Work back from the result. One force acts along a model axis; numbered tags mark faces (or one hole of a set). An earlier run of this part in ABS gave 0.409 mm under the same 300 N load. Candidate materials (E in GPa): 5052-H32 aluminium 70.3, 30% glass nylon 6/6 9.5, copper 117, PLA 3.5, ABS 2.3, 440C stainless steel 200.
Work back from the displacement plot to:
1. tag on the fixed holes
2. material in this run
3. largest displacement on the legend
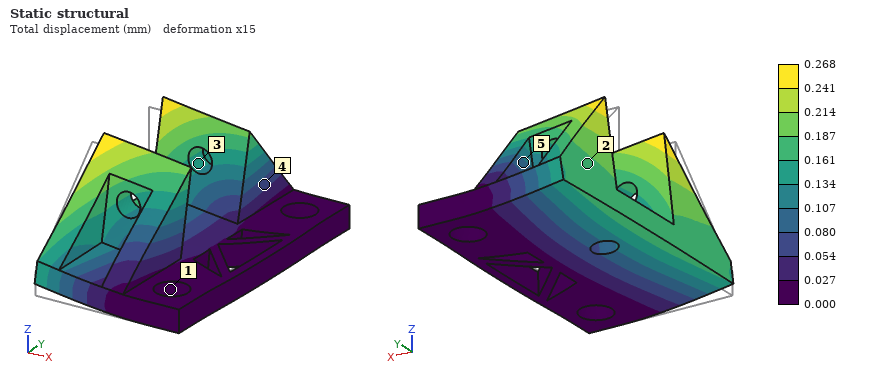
1
PLA
0.268 mm
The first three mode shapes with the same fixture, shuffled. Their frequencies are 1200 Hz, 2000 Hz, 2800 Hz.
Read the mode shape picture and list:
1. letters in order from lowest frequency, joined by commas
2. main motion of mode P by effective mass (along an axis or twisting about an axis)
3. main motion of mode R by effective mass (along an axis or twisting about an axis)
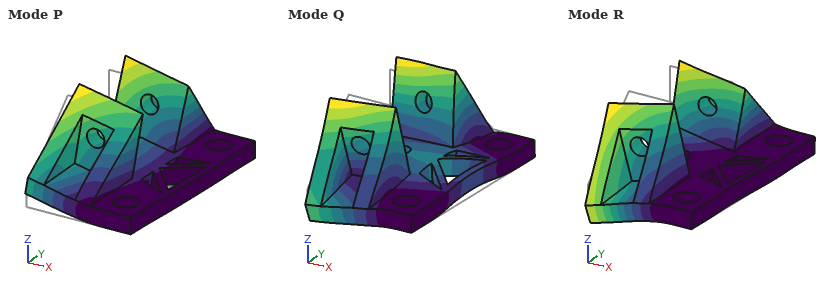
P, R, Q
along Z
twisting about X
